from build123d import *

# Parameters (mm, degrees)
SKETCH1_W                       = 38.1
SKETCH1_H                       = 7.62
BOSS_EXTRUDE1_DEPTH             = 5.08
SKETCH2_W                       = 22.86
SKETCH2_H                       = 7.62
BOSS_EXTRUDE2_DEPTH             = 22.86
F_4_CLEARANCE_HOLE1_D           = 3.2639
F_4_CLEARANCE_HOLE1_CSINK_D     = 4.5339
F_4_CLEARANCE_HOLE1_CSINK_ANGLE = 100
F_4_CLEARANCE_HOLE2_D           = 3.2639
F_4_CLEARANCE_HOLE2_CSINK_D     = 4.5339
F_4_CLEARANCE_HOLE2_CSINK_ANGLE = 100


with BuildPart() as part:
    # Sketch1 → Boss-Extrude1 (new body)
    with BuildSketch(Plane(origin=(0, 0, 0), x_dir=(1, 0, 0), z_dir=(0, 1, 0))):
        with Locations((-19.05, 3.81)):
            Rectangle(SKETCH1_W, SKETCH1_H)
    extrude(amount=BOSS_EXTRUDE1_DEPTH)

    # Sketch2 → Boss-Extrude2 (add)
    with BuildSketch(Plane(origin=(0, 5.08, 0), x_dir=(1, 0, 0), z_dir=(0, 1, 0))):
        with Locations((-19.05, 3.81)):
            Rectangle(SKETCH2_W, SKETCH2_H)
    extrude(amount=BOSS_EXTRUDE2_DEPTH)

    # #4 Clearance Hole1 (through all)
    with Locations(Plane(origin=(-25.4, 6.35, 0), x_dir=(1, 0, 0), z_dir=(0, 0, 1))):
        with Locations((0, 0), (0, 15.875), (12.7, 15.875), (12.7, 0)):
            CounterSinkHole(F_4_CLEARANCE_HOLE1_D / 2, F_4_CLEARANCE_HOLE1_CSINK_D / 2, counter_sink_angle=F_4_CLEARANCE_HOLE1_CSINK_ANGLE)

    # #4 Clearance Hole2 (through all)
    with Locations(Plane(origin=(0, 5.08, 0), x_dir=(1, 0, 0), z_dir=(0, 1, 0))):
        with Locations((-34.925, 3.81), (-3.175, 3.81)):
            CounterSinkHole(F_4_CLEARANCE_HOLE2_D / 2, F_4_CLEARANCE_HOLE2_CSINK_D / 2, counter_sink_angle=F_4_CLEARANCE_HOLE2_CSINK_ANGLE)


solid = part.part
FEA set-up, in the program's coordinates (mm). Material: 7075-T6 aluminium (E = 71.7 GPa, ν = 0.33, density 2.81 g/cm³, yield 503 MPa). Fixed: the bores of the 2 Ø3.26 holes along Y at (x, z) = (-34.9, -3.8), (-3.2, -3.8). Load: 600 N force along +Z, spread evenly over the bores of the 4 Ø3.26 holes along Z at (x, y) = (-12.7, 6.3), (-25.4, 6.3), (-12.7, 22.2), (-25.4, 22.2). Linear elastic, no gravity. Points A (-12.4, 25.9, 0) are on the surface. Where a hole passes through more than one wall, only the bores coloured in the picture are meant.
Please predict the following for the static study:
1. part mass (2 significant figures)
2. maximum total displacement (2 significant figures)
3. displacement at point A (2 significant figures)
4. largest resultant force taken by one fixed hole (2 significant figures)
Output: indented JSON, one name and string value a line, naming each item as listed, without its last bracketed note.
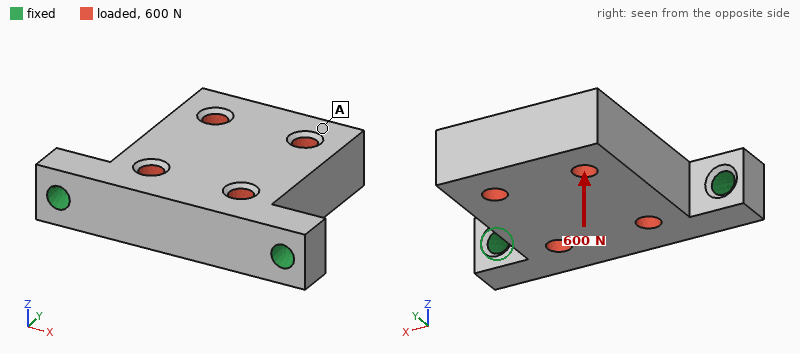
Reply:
{
  "part mass": "14 g",
  "maximum total displacement": "0.12 mm",
  "displacement at point A": "0.11 mm",
  "largest resultant force taken by one fixed hole": "300 N"
}
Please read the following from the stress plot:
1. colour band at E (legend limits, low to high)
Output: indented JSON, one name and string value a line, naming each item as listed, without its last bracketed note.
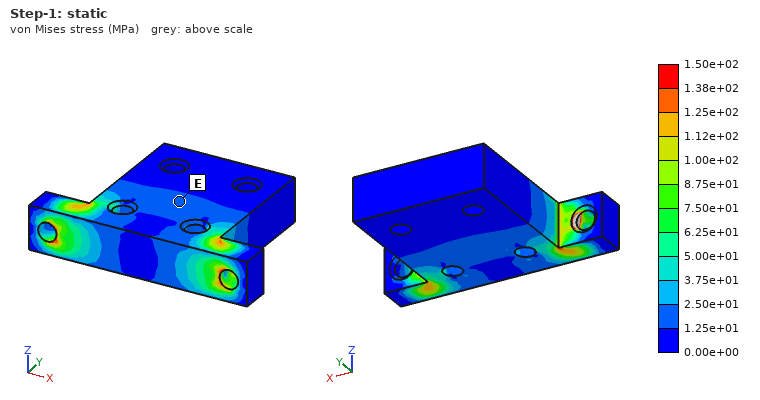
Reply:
{
  "colour band at E": "1.25e+01 to 2.50e+01 MPa"
}
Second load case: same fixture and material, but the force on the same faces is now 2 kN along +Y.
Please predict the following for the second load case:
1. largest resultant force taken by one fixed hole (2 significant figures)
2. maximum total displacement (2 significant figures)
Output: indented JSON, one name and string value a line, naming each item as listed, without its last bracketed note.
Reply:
{
  "largest resultant force taken by one fixed hole": "1.1 kN",
  "maximum total displacement": "17 µm"
}
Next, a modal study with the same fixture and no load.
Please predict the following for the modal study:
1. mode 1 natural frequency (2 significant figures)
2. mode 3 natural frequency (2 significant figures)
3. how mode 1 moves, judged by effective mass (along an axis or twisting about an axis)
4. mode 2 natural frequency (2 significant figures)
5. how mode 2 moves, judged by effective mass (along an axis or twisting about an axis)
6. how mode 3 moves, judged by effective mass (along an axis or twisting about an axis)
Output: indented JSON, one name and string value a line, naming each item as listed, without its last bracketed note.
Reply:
{
  "mode 1 natural frequency": "3900 Hz",
  "mode 3 natural frequency": "17 kHz",
  "how mode 1 moves, judged by effective mass": "along Z",
  "mode 2 natural frequency": "14 kHz",
  "how mode 2 moves, judged by effective mass": "along X",
  "how mode 3 moves, judged by effective mass": "twisting about Y"
}
